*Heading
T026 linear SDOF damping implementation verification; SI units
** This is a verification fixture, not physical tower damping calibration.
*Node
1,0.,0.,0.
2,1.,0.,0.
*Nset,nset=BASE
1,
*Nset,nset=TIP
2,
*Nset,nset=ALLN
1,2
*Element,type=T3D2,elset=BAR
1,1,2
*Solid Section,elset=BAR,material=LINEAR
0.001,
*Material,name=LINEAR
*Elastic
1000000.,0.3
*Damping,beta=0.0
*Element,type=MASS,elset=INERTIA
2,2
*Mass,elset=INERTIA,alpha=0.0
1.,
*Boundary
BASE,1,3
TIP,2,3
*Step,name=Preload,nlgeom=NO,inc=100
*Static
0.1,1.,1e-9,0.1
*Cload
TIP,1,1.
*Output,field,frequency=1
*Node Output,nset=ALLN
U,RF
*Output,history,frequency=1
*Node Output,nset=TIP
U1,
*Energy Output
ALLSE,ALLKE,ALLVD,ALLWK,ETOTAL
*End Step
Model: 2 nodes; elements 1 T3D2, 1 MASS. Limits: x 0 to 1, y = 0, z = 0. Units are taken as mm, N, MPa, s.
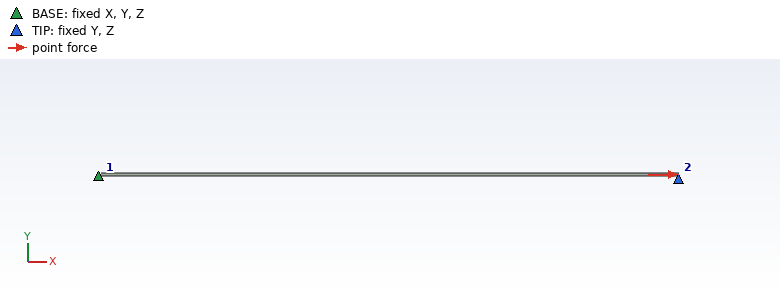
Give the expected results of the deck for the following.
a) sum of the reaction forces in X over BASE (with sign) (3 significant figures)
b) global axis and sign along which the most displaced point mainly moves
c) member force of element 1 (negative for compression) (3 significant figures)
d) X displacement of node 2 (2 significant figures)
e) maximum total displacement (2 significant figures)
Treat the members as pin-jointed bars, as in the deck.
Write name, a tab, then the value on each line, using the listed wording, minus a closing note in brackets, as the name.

sum of the reaction forces in X over BASE (with sign)	-1.00 N
global axis and sign along which the most displaced point mainly moves	+X
member force of element 1 (negative for compression)	1.00 N
X displacement of node 2	0.0010 mm
maximum total displacement	0.0010 mm
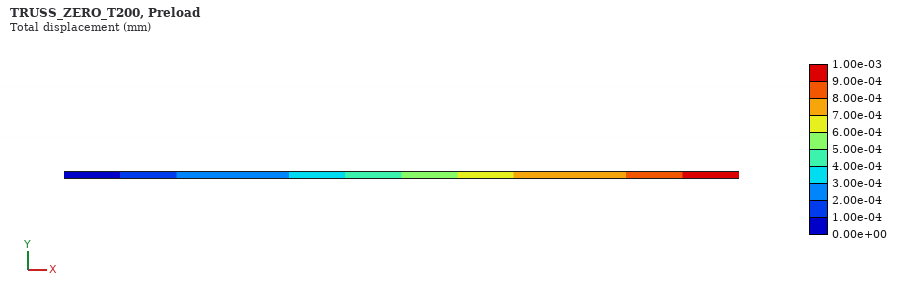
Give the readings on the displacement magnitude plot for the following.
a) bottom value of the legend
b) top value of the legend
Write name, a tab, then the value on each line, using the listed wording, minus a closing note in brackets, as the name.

bottom value of the legend	0.00e+00 mm
top value of the legend	1.00e-03 mm
